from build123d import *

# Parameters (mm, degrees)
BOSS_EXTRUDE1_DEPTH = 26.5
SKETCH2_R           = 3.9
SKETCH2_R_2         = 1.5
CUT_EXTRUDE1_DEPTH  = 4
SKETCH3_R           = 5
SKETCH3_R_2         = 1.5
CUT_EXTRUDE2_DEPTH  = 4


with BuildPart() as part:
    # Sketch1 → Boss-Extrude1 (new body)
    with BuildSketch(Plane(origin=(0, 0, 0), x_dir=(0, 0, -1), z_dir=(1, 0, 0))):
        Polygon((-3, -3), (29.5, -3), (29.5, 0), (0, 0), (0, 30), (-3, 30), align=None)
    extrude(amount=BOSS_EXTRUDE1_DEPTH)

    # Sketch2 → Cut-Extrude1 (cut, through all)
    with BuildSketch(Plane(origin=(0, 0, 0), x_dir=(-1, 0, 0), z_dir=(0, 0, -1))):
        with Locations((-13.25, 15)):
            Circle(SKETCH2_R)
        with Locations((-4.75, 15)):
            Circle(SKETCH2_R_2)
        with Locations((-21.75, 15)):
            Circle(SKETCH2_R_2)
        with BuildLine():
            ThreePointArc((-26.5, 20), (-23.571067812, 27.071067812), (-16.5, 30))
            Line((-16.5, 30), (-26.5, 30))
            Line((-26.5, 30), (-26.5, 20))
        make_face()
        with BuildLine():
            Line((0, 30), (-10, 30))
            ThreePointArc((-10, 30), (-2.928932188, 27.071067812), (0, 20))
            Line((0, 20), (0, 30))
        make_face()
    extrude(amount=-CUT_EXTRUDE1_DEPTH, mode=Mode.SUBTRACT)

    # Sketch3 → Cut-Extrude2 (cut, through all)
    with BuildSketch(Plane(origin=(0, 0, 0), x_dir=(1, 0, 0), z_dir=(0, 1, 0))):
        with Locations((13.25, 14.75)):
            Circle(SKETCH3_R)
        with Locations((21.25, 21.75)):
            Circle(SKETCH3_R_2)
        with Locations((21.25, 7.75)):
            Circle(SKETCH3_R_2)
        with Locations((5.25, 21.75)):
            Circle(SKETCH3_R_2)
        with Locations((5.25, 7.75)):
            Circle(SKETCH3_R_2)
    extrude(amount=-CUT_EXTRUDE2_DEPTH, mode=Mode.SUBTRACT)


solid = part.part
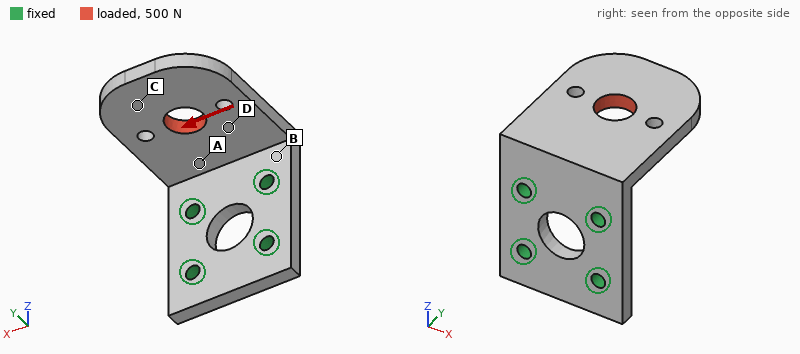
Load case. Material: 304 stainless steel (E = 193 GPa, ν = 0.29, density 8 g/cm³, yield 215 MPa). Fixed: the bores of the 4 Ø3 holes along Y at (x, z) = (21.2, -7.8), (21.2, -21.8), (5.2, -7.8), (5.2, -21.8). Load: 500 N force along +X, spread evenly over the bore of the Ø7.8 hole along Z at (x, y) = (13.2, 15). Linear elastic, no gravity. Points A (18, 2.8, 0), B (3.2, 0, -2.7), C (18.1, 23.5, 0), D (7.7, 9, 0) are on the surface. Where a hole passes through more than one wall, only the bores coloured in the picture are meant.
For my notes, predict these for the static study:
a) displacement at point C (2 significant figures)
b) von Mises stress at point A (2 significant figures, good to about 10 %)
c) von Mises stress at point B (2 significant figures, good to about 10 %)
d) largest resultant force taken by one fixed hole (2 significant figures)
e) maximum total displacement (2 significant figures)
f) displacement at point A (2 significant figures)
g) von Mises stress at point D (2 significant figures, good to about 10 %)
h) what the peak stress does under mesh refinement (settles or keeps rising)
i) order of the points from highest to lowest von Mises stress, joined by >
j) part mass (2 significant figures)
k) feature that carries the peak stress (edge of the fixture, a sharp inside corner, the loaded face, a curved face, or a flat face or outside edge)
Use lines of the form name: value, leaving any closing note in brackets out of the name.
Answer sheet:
displacement at point C: 37 µm
von Mises stress at point A: 49 MPa
von Mises stress at point B: 64 MPa
largest resultant force taken by one fixed hole: 570 N
maximum total displacement: 45 µm
displacement at point A: 9.0 µm
von Mises stress at point D: 23 MPa
what the peak stress does under mesh refinement: keeps rising
order of the points from highest to lowest von Mises stress, joined by >: B > A > D > C
part mass: 35 g
feature that carries the peak stress: edge of the fixture
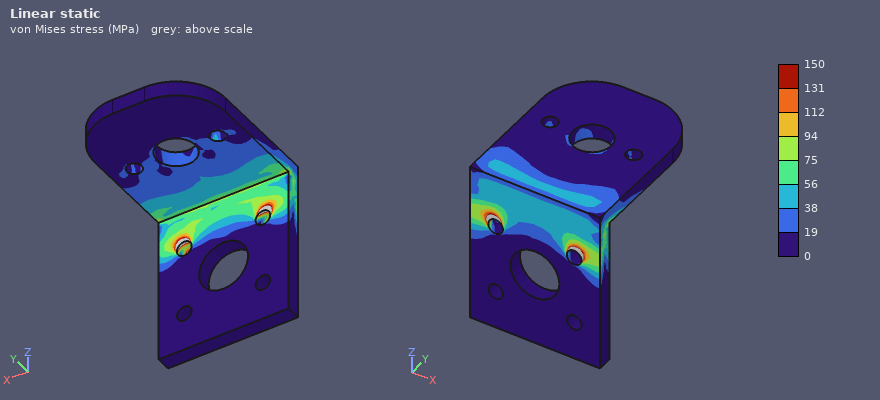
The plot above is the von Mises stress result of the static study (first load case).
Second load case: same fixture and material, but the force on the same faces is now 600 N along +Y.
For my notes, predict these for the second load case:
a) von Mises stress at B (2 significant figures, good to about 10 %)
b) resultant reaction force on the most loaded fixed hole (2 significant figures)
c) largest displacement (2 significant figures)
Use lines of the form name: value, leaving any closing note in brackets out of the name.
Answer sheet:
von Mises stress at B: 62 MPa
resultant reaction force on the most loaded fixed hole: 330 N
largest displacement: 71 µm
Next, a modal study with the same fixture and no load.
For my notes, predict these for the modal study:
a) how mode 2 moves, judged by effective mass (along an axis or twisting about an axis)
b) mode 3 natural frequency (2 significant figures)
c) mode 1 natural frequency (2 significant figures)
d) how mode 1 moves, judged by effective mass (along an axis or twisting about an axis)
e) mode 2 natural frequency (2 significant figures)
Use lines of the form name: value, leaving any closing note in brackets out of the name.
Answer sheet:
how mode 2 moves, judged by effective mass: along X
mode 3 natural frequency: 7100 Hz
mode 1 natural frequency: 1800 Hz
how mode 1 moves, judged by effective mass: along Z
mode 2 natural frequency: 4700 Hz
